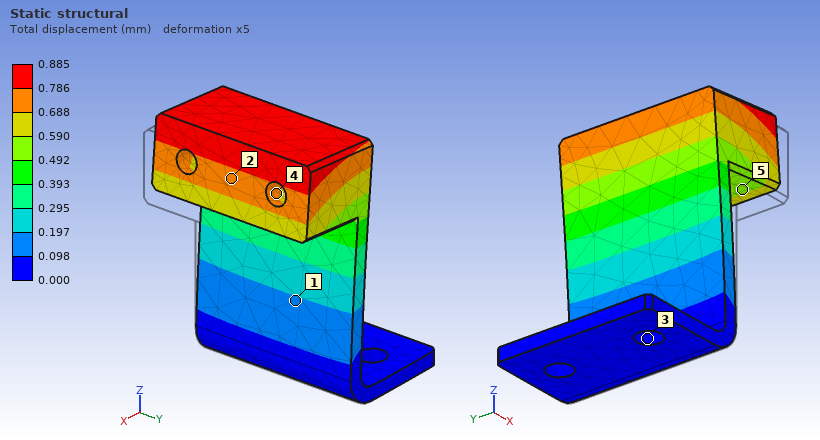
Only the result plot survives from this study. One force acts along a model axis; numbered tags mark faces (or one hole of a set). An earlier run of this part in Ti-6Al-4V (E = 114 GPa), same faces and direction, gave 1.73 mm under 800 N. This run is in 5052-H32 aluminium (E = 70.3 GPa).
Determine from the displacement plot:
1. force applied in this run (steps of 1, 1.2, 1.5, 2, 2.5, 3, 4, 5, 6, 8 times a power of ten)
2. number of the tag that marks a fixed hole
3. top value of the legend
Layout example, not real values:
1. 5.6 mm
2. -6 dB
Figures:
1. 250 N
2. 3
3. 0.885 mm
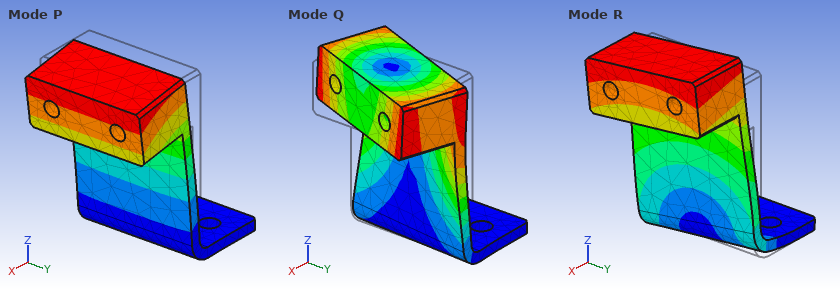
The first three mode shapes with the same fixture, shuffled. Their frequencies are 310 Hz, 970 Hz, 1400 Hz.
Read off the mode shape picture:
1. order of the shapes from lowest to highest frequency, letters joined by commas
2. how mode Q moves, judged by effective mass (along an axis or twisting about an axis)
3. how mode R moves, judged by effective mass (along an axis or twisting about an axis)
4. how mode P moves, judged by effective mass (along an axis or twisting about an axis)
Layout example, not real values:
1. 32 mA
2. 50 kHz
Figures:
1. P, R, Q
2. twisting about Z
3. along Y
4. along X
